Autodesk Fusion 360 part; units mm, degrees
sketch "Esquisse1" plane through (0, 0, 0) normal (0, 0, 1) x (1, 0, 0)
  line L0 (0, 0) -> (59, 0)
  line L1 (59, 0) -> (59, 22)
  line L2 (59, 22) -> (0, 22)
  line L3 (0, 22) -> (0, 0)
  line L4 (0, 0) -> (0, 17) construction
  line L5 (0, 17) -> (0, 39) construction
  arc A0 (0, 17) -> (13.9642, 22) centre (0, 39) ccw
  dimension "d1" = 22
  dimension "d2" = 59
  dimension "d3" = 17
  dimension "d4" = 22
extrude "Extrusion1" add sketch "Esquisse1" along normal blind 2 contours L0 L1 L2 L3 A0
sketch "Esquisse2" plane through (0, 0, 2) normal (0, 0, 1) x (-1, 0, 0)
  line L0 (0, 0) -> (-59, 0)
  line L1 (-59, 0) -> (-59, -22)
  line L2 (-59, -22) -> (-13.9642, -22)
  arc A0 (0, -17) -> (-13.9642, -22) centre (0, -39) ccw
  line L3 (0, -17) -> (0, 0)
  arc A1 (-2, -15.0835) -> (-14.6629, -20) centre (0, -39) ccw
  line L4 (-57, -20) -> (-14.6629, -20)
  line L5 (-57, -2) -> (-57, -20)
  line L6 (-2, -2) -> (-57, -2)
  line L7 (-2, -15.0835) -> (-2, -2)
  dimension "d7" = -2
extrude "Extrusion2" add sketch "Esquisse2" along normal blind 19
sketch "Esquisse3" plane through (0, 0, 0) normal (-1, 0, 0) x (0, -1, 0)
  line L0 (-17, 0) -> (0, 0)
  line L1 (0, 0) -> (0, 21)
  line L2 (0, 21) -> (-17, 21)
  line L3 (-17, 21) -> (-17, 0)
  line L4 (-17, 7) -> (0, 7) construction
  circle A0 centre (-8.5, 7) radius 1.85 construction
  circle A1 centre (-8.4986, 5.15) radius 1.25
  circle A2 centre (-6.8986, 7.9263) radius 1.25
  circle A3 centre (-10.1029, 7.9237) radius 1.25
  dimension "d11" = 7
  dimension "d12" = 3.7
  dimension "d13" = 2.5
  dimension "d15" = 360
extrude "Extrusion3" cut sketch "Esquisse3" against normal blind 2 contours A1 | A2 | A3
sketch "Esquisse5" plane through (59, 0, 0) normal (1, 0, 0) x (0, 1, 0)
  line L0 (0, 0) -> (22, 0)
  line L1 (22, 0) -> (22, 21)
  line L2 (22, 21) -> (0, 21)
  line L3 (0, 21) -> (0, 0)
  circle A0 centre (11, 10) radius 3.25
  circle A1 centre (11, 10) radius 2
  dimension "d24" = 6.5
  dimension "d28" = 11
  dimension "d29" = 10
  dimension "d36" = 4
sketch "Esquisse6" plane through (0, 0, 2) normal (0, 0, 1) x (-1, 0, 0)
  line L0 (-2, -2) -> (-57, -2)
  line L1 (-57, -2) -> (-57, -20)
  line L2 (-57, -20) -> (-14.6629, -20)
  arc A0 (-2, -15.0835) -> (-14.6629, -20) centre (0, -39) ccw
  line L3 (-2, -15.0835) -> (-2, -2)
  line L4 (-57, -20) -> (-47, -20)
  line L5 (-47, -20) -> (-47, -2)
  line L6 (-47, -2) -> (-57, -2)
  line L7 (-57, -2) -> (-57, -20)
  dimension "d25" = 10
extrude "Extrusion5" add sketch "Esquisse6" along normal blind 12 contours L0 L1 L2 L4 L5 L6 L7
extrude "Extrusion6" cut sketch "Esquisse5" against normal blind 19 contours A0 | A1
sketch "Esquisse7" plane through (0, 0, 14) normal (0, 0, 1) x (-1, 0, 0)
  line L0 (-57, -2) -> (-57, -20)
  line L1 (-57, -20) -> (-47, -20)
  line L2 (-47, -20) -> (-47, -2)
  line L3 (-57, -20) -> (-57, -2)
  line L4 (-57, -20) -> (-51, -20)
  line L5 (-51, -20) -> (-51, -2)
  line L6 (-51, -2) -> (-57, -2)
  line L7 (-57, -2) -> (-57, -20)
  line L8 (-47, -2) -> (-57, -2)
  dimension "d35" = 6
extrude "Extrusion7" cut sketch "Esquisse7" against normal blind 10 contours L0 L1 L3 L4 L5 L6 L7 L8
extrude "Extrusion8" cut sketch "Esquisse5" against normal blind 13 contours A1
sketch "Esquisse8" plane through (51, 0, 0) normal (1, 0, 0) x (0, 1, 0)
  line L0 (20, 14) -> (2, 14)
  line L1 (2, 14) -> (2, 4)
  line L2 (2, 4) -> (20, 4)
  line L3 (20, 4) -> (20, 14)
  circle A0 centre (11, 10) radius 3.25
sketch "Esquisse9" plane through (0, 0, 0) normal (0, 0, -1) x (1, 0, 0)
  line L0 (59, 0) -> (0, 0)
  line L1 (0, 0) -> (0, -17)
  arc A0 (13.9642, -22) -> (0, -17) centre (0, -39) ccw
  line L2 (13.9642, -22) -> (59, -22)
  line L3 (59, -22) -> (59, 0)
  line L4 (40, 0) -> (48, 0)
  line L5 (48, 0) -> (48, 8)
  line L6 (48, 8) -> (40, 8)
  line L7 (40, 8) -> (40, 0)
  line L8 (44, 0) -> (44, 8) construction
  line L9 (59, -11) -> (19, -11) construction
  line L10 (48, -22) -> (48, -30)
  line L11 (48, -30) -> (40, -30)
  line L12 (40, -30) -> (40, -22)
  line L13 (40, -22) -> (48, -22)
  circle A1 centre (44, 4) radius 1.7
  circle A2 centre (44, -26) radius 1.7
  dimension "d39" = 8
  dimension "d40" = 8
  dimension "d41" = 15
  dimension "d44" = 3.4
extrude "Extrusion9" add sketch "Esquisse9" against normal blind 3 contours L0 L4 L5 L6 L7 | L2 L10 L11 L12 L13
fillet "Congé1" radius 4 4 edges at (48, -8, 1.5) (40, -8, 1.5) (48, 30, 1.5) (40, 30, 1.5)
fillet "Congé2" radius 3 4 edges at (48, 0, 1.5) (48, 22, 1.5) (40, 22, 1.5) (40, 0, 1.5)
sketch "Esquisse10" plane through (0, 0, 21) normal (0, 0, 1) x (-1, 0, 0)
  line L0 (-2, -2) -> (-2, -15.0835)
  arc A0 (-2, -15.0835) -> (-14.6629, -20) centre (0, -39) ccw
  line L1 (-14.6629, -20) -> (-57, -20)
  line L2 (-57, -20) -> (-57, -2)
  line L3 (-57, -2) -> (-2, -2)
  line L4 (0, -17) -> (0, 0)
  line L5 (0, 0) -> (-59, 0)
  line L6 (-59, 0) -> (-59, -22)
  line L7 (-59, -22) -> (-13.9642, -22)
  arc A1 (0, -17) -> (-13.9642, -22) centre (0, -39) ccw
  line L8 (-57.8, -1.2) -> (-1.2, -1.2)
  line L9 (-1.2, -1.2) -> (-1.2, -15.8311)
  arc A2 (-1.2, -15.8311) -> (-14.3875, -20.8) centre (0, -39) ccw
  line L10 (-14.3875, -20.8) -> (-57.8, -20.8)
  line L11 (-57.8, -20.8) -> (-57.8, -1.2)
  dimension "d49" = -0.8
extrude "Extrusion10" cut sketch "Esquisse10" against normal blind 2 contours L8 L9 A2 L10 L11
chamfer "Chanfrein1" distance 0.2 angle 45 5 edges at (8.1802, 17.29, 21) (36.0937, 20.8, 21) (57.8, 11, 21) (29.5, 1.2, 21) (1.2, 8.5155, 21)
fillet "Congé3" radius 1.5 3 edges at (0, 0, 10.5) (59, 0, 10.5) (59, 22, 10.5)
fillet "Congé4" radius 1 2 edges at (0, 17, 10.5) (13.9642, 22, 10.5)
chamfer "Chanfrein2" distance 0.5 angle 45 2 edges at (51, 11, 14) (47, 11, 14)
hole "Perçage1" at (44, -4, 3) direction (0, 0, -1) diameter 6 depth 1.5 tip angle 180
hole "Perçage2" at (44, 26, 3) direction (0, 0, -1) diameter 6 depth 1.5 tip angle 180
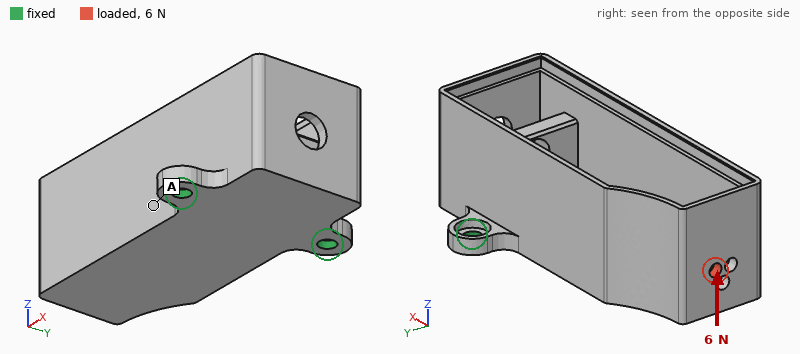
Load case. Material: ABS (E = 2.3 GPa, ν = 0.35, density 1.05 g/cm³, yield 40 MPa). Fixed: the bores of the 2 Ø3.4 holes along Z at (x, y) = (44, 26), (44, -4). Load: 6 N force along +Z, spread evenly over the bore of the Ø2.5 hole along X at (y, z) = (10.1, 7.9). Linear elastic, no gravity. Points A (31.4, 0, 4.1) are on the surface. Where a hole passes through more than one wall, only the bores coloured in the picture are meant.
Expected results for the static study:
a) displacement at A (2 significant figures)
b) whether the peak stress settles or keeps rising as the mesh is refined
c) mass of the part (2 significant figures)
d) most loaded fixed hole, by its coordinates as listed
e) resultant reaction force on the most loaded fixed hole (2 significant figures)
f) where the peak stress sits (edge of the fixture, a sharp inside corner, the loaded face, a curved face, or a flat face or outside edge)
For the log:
0.21 mm
keeps rising
9.5 g
(44, -4)
3.3 N
edge of the fixture
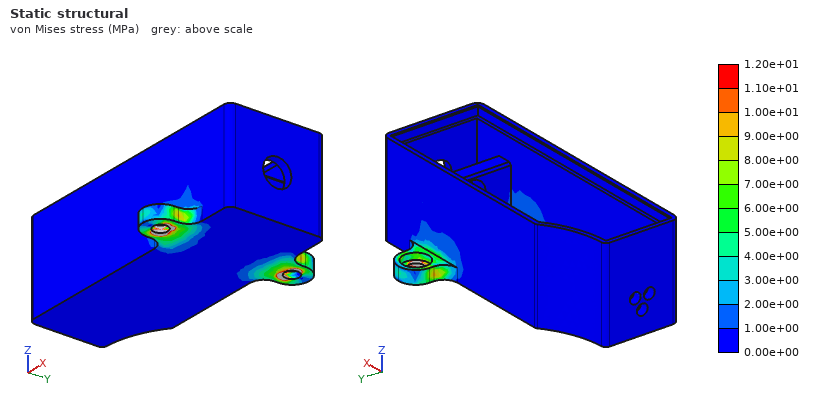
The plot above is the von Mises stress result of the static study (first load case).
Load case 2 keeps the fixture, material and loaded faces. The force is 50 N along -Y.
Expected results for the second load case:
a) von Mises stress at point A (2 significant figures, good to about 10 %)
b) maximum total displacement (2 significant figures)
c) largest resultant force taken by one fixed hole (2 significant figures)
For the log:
4.8 MPa
0.87 mm
81 N
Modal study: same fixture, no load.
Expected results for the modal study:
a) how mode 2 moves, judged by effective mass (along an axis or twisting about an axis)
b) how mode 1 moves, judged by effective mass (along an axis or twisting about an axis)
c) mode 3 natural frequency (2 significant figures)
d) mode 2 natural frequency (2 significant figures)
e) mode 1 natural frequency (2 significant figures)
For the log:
along Y
along Z
1700 Hz
830 Hz
280 Hz
